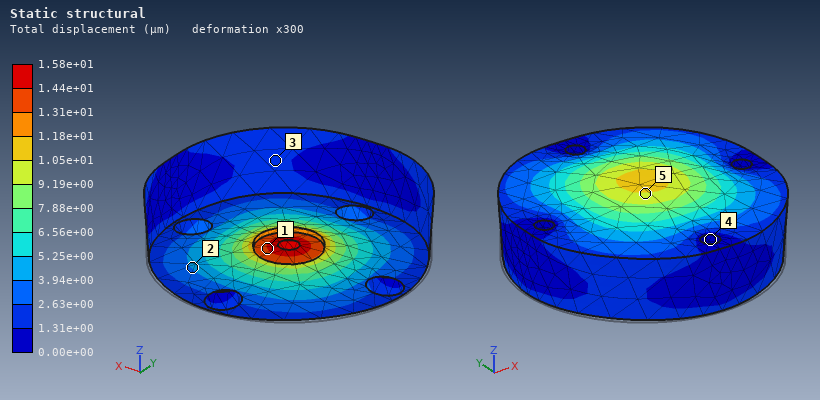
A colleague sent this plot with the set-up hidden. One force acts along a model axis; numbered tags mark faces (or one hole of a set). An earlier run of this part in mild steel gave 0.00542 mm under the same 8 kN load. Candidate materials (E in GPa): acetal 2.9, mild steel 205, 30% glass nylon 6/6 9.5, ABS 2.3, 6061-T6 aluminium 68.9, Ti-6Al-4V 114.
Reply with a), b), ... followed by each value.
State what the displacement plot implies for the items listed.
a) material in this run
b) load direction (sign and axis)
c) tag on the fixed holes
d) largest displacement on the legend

a) 6061-T6 aluminium
b) +Z
c) 4
d) 1.58e+01 µm
